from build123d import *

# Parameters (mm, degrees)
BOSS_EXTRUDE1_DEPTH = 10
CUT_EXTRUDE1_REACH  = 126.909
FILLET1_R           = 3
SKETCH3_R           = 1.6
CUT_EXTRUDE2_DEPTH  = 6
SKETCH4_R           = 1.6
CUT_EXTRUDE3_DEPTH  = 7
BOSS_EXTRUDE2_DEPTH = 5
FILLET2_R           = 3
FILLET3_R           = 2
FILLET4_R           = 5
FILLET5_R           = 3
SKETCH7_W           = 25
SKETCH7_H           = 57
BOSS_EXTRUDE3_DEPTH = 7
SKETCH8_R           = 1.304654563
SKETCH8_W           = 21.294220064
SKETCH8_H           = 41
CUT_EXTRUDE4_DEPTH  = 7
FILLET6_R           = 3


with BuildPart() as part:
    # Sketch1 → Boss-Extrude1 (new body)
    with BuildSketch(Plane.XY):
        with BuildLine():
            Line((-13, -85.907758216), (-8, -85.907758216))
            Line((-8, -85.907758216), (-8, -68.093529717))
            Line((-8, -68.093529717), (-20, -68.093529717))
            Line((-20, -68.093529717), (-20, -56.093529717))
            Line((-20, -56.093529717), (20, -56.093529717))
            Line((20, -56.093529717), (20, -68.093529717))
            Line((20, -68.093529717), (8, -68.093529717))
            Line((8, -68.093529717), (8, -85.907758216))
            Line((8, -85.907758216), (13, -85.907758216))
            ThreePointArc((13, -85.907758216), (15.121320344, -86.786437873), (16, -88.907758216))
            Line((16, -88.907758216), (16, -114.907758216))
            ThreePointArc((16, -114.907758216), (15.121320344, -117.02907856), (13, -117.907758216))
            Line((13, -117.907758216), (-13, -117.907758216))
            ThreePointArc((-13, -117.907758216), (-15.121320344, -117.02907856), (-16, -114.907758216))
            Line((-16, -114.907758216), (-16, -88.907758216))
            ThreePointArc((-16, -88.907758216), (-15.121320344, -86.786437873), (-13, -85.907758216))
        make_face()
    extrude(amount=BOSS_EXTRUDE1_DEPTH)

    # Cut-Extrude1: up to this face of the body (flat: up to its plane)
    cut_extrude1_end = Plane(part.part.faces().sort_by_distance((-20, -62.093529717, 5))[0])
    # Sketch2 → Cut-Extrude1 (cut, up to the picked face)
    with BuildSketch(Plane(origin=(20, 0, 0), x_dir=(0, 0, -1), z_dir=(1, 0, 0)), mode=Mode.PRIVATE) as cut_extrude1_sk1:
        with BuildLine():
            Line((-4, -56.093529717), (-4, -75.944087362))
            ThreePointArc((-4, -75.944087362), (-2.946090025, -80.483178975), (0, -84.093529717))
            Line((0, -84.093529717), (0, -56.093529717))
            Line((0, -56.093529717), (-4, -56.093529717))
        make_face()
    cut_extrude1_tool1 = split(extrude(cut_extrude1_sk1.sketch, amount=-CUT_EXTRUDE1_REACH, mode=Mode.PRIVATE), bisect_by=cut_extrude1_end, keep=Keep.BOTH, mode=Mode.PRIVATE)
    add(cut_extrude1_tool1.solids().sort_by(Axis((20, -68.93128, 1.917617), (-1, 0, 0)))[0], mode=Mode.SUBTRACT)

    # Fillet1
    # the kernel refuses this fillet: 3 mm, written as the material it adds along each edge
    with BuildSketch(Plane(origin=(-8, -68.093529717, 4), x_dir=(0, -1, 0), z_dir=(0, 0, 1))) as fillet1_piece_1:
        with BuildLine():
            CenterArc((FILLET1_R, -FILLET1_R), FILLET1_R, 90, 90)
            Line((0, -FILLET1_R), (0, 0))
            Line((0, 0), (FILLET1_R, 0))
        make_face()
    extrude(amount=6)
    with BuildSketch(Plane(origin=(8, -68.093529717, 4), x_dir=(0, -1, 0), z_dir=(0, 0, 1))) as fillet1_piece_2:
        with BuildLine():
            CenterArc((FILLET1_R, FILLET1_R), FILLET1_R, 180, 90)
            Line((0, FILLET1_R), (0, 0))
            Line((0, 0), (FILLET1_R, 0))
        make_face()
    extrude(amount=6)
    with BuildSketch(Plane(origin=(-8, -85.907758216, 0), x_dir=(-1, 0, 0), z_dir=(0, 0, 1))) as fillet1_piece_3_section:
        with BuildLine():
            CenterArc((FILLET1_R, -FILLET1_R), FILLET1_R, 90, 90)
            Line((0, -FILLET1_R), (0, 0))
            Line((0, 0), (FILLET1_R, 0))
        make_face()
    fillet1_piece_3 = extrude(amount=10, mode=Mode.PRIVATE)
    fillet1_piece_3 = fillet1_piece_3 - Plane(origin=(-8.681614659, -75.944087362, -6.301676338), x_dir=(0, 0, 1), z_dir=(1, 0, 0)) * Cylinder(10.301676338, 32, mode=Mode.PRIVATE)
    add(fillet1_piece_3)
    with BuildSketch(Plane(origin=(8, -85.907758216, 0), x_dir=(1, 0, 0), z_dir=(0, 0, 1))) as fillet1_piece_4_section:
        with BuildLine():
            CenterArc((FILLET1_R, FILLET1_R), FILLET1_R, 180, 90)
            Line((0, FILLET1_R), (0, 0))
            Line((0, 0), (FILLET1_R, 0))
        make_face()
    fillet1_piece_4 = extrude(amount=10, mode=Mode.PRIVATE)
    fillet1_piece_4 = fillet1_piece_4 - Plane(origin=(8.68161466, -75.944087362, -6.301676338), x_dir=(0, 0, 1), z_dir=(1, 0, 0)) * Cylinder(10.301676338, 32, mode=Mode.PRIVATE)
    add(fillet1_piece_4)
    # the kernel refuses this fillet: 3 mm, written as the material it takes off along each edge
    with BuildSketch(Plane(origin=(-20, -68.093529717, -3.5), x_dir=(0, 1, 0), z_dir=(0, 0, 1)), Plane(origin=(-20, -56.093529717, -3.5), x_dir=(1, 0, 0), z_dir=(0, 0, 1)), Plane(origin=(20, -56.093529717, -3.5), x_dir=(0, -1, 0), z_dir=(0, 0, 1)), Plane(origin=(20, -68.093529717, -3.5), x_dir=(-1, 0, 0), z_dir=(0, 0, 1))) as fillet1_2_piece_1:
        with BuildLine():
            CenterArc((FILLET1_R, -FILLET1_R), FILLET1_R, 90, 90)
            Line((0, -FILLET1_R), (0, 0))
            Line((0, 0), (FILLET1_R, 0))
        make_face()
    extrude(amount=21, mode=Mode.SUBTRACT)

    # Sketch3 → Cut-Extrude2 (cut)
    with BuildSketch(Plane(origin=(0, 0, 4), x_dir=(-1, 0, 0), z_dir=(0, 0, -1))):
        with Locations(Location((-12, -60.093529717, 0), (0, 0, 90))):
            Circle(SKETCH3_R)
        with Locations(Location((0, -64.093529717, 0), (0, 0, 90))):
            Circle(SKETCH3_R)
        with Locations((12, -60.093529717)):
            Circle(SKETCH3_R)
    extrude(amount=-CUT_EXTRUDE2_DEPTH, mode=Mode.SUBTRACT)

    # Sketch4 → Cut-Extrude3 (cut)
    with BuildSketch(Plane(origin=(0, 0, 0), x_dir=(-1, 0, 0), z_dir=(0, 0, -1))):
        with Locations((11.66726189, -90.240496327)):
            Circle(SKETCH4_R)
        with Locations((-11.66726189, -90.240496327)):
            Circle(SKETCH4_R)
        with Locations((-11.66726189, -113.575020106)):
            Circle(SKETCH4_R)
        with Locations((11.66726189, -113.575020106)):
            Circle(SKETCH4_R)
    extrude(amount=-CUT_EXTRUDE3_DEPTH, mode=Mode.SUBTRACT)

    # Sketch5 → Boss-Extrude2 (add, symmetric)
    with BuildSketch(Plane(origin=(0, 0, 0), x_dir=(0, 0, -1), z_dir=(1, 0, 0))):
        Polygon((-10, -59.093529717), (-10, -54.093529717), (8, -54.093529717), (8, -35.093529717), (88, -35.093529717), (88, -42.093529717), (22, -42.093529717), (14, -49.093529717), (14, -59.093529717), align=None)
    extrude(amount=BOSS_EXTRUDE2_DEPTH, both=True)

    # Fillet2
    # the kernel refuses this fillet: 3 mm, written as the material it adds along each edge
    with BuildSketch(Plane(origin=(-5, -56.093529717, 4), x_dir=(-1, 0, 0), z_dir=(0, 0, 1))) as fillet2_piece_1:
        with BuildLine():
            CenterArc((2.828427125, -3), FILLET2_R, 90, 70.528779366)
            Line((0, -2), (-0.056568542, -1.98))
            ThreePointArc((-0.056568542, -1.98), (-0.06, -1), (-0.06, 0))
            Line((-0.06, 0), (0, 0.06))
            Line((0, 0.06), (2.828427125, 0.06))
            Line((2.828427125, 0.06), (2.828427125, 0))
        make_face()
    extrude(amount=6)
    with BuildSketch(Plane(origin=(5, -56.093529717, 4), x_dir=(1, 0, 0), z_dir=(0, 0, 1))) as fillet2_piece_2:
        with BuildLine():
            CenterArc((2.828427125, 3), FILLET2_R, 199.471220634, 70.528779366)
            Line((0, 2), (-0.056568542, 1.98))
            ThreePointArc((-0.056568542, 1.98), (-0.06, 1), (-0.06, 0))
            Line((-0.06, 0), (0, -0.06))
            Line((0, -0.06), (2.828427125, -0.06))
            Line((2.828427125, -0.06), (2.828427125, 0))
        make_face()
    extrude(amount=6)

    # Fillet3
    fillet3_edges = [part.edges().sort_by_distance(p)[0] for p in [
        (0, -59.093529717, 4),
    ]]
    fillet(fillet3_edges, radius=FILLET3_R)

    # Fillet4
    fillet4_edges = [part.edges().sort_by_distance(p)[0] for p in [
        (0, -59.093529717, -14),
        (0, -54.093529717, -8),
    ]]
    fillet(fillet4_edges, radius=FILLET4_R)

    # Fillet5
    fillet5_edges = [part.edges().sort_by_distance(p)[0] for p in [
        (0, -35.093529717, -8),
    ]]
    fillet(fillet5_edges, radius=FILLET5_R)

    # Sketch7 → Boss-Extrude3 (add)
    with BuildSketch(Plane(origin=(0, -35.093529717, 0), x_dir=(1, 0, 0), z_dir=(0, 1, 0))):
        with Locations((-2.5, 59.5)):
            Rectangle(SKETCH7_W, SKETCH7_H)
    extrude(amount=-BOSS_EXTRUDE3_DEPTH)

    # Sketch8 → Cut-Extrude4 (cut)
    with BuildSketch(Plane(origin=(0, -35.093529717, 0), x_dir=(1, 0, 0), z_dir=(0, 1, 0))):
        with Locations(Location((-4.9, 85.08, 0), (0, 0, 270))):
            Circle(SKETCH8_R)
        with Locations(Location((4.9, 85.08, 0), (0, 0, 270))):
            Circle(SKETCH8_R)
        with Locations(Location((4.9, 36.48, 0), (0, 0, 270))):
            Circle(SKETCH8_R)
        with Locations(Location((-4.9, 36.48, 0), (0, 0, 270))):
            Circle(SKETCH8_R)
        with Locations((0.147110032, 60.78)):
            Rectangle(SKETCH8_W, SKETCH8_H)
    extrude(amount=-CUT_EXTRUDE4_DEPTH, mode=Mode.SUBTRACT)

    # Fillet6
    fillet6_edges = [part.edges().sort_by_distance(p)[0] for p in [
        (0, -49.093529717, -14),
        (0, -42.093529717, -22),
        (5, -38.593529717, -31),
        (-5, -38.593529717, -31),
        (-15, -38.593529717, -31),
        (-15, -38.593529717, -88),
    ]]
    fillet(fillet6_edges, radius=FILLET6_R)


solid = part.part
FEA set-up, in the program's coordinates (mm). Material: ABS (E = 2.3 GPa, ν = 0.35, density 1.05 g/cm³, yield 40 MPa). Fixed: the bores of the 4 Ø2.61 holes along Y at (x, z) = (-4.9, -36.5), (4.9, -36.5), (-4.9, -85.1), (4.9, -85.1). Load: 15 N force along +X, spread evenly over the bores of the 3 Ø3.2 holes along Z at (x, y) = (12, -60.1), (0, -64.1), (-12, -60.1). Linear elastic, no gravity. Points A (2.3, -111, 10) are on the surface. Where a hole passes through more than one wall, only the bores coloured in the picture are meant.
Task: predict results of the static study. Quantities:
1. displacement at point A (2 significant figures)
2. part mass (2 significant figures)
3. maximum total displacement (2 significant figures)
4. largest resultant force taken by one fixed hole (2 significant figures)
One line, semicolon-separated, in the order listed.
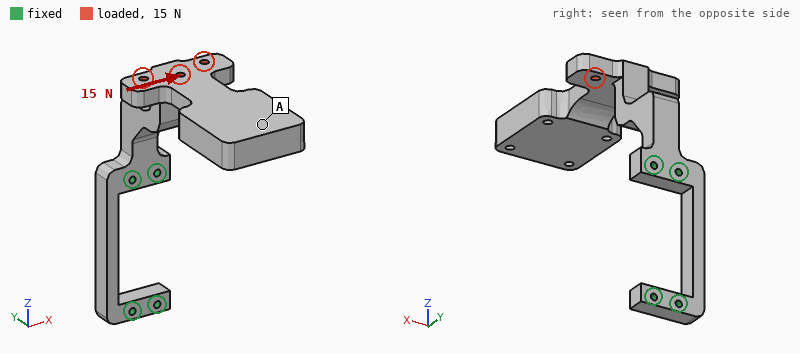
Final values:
1.1 mm; 23 g; 1.2 mm; 64 N
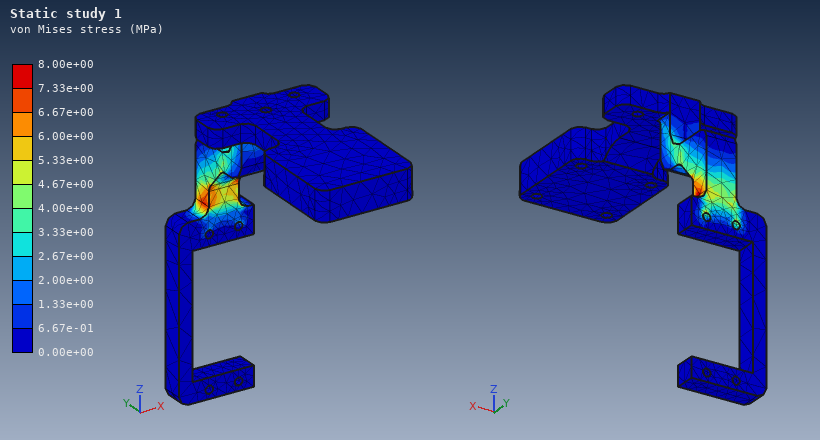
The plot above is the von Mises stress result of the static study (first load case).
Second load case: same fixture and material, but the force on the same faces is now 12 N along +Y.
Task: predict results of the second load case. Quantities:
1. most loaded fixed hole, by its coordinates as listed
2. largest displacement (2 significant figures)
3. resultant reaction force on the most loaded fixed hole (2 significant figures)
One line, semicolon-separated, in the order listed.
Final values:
(-4.9, -36.5); 1.5 mm; 6.6 N
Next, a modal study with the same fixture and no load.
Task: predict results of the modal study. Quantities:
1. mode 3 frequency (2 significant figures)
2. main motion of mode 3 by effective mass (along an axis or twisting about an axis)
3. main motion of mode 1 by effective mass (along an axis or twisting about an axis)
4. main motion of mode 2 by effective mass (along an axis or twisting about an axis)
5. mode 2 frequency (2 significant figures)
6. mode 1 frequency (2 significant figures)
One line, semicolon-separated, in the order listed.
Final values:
340 Hz; along Y; along Z; along X; 95 Hz; 81 Hz
